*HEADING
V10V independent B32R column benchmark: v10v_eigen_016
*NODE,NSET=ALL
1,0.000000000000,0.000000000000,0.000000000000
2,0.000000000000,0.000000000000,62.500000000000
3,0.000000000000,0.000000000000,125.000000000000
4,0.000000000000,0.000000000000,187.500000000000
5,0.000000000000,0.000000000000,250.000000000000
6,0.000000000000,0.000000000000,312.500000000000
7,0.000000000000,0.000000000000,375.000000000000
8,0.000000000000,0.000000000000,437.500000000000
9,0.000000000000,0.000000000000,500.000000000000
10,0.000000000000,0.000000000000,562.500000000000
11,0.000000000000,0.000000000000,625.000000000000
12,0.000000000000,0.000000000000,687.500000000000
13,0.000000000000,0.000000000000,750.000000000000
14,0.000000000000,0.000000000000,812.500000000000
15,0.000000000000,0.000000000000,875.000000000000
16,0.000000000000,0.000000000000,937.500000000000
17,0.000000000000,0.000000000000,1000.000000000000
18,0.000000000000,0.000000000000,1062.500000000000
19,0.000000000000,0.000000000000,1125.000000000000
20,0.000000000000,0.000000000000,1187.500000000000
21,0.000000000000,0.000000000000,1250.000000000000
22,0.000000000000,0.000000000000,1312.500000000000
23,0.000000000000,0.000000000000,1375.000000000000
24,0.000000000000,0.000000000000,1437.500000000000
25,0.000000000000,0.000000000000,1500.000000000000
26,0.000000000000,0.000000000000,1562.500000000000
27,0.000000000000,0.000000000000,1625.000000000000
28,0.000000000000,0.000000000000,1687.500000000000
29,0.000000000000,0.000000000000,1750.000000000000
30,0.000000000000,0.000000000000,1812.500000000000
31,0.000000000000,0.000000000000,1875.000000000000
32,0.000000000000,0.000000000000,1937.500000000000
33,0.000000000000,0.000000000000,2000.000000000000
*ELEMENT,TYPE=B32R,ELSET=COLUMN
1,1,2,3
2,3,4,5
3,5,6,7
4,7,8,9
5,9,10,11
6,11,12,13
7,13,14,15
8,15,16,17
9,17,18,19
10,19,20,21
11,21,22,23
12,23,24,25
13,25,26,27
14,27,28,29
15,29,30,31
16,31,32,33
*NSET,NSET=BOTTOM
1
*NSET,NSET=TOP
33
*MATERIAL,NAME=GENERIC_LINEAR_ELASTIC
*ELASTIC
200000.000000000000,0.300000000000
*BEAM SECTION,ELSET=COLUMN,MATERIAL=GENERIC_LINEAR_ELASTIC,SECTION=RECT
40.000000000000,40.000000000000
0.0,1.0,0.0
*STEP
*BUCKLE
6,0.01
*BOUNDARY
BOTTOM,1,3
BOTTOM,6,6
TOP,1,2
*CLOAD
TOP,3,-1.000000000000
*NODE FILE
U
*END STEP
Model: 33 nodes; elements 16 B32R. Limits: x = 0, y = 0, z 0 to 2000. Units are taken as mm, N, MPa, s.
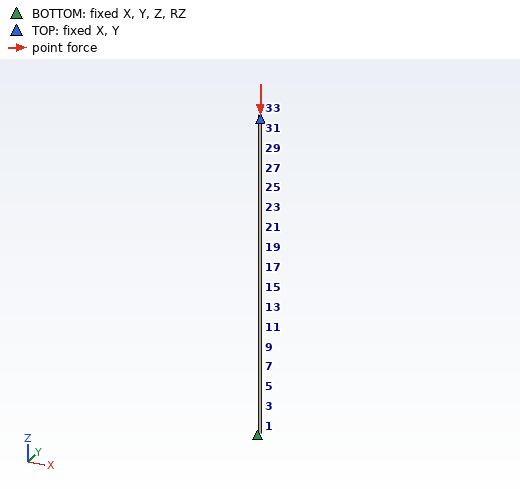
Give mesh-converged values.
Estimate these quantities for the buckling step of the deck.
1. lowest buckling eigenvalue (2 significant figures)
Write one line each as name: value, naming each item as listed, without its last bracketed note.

lowest buckling eigenvalue: 1.1e+05
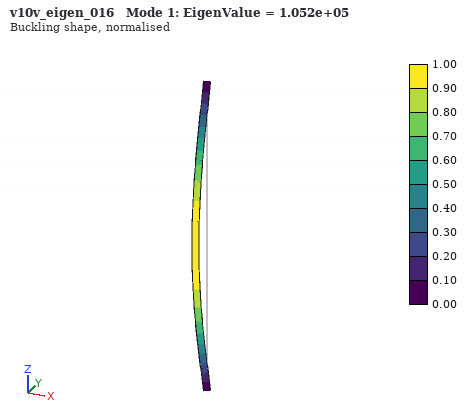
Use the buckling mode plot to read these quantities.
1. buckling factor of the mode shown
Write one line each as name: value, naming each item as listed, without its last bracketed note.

buckling factor of the mode shown: 1.052e+05
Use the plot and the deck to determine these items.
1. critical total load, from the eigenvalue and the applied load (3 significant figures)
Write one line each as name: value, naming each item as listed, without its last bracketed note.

critical total load, from the eigenvalue and the applied load: 1.05e+05 N
